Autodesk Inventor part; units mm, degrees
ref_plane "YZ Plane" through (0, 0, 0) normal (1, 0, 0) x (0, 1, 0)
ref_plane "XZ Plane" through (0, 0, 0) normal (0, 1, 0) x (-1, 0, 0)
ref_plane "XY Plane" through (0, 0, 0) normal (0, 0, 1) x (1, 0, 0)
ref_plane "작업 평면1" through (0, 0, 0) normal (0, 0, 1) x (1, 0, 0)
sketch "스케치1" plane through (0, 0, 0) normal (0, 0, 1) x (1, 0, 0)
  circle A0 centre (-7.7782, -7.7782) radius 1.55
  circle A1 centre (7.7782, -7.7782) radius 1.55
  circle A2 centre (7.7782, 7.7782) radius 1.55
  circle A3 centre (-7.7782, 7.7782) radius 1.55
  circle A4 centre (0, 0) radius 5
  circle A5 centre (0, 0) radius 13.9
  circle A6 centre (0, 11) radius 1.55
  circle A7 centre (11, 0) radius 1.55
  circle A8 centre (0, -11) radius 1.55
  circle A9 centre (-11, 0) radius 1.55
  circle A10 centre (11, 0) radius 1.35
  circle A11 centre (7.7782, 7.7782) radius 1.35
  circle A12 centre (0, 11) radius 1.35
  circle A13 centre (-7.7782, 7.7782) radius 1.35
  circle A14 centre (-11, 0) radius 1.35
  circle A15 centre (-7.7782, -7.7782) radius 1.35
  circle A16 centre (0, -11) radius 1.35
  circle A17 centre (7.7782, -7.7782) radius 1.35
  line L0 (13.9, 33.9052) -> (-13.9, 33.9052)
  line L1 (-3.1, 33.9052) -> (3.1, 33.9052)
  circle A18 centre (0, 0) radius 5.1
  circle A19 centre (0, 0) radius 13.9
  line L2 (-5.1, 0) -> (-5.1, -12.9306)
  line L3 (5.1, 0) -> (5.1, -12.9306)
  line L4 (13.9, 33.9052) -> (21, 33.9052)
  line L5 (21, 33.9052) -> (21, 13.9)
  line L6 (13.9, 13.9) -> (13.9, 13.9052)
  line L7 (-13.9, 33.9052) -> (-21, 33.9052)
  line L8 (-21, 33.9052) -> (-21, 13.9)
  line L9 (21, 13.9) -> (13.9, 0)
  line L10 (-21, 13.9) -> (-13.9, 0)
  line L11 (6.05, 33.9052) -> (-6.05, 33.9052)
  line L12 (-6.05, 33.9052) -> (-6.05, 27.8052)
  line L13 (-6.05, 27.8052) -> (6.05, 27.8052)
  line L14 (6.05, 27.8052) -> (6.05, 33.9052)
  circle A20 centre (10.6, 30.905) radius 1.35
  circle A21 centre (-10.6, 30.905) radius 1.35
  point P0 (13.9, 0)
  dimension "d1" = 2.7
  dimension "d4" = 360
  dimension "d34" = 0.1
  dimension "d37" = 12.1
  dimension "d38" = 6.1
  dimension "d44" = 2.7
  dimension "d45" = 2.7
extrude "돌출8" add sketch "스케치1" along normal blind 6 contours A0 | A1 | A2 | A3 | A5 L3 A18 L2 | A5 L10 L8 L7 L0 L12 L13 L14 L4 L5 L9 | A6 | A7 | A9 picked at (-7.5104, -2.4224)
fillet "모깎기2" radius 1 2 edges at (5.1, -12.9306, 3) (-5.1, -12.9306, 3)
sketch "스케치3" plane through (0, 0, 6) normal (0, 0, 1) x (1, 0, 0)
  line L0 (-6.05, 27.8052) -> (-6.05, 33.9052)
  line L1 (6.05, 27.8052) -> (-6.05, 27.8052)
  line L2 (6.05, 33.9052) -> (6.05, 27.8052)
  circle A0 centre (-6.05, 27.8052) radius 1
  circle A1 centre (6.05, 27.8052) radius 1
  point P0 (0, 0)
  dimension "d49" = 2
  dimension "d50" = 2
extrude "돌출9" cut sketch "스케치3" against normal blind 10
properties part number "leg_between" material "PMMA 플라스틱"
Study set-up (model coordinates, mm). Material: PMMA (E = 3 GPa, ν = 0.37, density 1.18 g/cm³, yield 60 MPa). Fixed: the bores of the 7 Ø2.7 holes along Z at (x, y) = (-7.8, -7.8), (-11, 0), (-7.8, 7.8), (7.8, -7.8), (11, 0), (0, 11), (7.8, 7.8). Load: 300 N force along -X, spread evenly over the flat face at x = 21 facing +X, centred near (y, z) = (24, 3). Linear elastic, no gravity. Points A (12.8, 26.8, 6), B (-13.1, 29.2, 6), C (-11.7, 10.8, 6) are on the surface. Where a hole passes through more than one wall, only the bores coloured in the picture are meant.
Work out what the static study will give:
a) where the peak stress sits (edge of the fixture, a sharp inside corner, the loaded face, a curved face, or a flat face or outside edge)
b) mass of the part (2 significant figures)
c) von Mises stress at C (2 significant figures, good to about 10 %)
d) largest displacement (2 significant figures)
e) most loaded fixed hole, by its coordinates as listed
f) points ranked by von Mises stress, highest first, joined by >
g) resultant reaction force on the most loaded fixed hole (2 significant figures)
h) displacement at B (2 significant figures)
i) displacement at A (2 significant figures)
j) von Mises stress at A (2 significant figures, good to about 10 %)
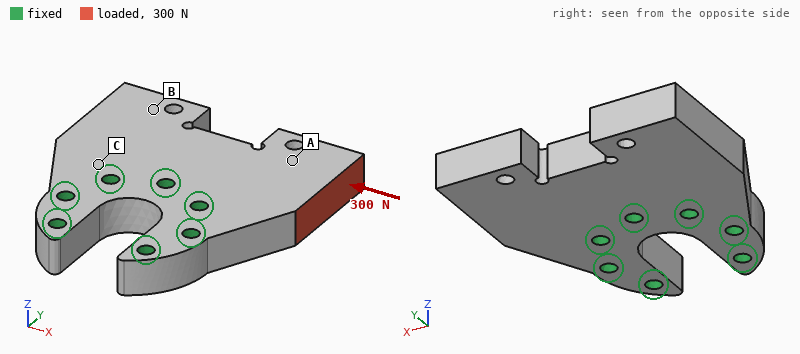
a curved face
9.3 g
2.1 MPa
99 µm
(0, 11)
A > C > B
210 N
33 µm
57 µm
3.7 MPa
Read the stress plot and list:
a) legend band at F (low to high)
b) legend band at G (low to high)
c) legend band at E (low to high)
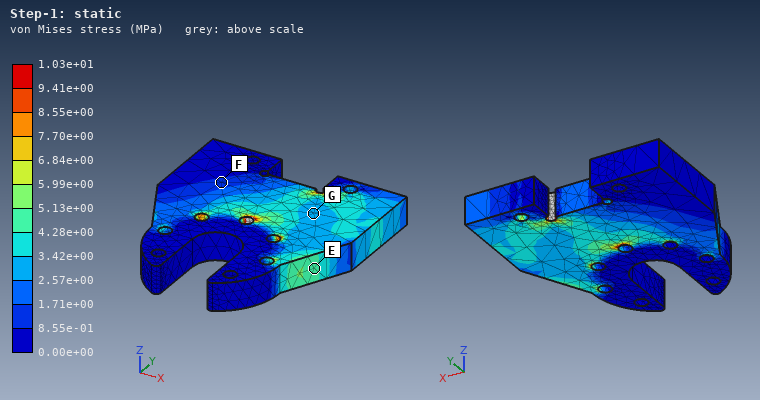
8.55e-01 to 1.71e+00 MPa
2.57e+00 to 3.42e+00 MPa
4.28e+00 to 5.13e+00 MPa
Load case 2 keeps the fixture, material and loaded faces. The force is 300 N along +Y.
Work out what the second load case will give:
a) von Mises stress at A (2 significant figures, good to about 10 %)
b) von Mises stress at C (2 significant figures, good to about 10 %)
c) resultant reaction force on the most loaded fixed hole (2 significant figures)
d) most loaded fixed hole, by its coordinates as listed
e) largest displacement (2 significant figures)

2.2 MPa
1.5 MPa
220 N
(7.8, 7.8)
0.13 mm
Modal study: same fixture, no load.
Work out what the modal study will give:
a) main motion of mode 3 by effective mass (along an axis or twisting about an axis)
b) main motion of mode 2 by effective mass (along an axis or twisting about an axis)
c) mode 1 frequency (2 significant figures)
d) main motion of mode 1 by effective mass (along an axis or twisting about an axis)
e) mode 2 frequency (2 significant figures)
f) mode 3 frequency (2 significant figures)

along X
twisting about Y
2500 Hz
along Z
2700 Hz
5800 Hz
